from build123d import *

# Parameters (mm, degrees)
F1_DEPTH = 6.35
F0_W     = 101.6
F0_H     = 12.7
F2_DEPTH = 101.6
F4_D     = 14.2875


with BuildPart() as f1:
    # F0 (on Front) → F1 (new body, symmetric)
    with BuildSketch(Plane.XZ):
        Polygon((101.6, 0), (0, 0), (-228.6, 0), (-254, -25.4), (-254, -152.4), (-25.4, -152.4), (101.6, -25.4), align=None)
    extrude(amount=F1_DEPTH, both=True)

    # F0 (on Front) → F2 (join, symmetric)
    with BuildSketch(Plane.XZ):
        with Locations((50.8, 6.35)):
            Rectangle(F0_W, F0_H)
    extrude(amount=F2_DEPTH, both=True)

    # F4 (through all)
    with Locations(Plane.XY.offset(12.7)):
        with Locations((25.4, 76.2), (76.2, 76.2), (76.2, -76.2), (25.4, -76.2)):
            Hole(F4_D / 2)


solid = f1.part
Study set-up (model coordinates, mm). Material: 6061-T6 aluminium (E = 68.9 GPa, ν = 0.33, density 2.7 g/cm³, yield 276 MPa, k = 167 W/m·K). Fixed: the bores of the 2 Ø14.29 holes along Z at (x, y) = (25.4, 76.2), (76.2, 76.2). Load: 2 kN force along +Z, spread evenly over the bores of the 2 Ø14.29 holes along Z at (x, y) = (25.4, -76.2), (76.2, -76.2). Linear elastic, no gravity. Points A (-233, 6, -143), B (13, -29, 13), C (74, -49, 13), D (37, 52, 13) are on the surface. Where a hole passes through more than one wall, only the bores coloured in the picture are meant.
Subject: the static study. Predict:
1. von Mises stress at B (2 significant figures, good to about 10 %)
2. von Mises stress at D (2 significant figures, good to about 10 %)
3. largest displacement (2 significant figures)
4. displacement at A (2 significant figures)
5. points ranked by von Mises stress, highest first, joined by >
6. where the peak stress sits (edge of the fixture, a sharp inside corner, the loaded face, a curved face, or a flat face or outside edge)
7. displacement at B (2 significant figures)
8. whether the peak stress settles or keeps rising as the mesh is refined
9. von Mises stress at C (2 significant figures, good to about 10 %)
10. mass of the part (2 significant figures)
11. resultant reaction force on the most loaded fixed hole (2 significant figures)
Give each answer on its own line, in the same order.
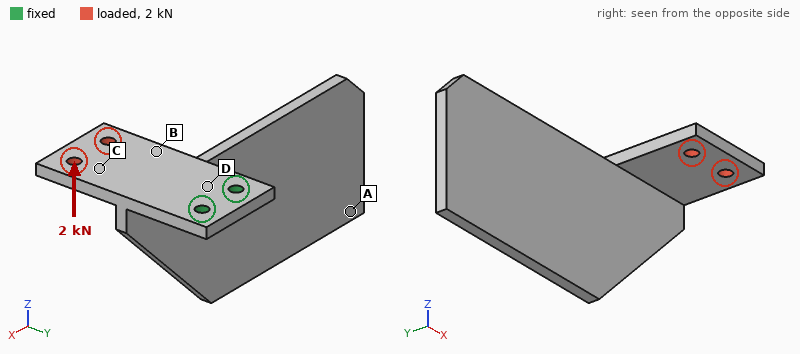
33 MPa
84 MPa
2.2 mm
2.0 mm
D > B > C > A
edge of the fixture
0.96 mm
keeps rising
19 MPa
2.3 kg
1.0 kN
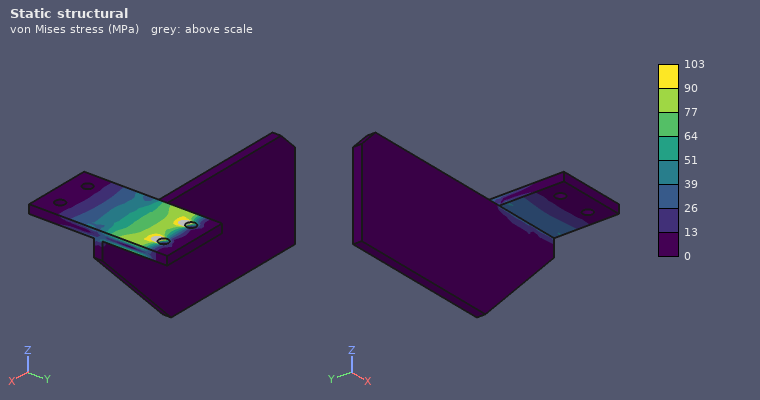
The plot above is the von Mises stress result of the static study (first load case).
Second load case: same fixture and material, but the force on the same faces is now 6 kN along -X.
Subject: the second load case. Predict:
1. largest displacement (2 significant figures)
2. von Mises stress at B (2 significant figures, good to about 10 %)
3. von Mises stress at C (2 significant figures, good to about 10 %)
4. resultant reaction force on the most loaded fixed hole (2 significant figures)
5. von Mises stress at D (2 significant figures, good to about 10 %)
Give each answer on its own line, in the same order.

0.28 mm
11 MPa
11 MPa
15 kN
22 MPa
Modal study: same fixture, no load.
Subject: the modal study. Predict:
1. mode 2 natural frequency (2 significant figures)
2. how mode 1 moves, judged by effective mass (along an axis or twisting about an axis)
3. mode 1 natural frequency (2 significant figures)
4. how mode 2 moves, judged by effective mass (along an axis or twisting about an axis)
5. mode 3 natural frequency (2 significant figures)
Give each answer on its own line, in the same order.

130 Hz
along Y
87 Hz
along Z
220 Hz
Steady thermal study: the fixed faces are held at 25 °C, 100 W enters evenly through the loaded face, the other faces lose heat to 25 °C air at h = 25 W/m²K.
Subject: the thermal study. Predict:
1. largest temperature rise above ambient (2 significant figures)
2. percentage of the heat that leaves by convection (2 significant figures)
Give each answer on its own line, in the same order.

52 K
48 %
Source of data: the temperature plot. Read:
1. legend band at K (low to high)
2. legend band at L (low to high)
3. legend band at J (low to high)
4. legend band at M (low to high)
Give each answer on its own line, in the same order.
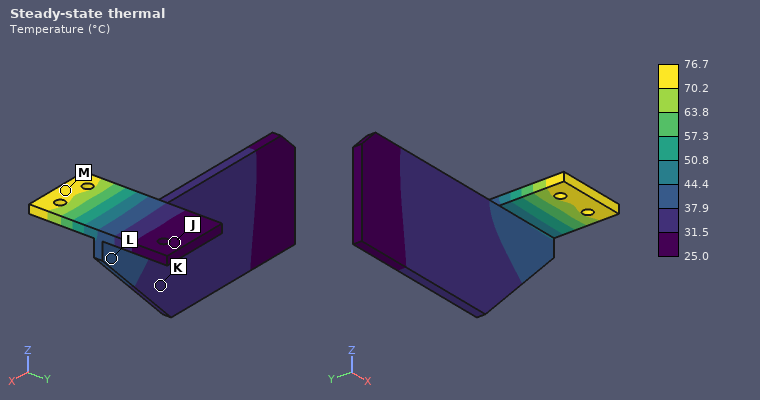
31.5 to 37.9 °C
37.9 to 44.4 °C
25.0 to 31.5 °C
70.2 to 76.7 °C
